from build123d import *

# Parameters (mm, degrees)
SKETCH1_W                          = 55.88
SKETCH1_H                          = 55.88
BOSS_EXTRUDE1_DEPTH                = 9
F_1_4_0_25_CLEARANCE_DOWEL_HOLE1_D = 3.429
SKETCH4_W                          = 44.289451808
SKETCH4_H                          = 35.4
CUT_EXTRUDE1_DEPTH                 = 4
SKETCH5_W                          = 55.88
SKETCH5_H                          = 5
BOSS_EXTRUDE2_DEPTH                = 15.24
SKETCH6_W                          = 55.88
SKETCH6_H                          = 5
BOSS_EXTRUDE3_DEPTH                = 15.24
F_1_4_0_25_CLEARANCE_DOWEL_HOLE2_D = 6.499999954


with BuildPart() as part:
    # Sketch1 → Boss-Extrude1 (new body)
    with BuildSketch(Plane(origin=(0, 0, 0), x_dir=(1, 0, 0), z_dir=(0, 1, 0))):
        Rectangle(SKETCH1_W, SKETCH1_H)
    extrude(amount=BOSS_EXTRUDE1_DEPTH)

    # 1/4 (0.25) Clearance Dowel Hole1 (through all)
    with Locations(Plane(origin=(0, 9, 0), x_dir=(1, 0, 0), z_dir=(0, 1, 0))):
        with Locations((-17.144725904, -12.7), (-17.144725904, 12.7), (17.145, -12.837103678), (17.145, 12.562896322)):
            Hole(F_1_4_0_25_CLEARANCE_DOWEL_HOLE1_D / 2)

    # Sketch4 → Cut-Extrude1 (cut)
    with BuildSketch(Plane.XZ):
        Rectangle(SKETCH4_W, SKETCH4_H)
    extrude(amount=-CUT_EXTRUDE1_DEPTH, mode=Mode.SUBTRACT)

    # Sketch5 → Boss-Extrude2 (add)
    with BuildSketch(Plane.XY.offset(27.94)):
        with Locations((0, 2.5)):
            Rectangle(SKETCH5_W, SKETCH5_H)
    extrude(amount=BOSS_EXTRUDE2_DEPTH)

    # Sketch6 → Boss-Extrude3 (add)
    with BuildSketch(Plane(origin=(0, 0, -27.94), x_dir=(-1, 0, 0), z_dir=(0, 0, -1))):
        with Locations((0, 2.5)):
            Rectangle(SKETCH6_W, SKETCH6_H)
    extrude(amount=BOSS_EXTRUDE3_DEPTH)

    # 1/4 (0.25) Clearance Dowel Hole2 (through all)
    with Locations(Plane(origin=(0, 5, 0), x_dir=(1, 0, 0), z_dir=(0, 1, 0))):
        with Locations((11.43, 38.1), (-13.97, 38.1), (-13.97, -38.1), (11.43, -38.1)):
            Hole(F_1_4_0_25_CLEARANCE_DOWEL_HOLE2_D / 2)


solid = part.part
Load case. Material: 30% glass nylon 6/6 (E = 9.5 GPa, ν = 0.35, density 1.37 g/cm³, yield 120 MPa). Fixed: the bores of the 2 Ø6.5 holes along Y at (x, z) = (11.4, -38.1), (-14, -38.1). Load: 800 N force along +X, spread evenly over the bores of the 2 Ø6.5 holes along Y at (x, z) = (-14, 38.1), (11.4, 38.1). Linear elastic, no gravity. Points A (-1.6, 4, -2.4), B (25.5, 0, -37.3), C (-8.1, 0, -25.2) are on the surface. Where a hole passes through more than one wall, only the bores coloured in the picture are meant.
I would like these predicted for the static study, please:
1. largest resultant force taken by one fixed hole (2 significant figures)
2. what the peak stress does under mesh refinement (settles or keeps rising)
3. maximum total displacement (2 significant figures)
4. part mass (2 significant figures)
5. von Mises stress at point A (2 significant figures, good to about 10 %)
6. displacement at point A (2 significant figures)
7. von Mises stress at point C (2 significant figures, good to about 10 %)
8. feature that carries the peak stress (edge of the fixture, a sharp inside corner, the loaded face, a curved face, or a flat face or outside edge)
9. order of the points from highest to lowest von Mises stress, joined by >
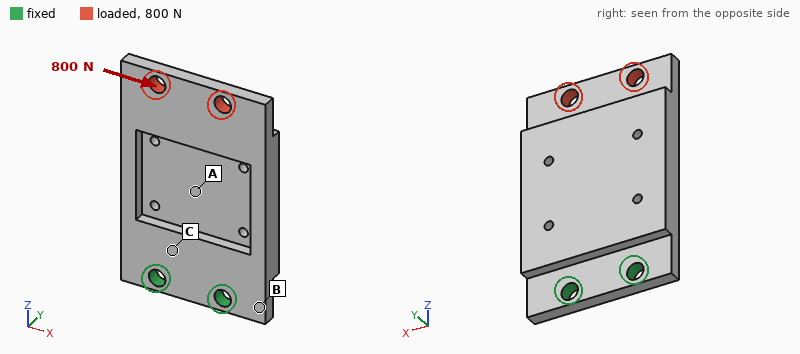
2.0 kN
keeps rising
0.73 mm
40 g
17 MPa
0.17 mm
30 MPa
edge of the fixture
C > A > B
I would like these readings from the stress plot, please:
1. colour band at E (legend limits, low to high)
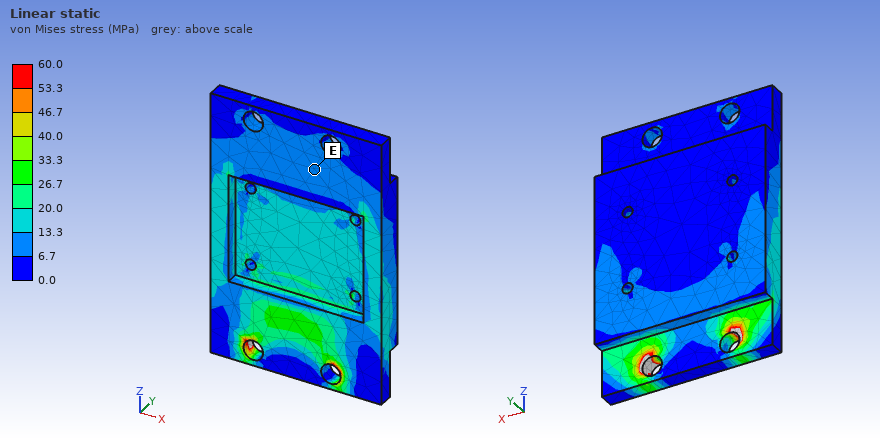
6.7 to 13.3 MPa
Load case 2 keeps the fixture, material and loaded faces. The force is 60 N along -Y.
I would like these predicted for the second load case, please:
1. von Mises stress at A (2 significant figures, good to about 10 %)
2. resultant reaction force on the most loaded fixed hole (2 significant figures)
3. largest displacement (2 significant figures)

4.2 MPa
53 N
1.1 mm
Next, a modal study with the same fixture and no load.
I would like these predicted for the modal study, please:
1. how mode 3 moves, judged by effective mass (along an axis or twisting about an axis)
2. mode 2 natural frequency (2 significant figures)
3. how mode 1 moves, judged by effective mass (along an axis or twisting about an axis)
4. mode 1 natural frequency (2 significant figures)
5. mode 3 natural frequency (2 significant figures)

along X
1100 Hz
along Y
370 Hz
2100 Hz
